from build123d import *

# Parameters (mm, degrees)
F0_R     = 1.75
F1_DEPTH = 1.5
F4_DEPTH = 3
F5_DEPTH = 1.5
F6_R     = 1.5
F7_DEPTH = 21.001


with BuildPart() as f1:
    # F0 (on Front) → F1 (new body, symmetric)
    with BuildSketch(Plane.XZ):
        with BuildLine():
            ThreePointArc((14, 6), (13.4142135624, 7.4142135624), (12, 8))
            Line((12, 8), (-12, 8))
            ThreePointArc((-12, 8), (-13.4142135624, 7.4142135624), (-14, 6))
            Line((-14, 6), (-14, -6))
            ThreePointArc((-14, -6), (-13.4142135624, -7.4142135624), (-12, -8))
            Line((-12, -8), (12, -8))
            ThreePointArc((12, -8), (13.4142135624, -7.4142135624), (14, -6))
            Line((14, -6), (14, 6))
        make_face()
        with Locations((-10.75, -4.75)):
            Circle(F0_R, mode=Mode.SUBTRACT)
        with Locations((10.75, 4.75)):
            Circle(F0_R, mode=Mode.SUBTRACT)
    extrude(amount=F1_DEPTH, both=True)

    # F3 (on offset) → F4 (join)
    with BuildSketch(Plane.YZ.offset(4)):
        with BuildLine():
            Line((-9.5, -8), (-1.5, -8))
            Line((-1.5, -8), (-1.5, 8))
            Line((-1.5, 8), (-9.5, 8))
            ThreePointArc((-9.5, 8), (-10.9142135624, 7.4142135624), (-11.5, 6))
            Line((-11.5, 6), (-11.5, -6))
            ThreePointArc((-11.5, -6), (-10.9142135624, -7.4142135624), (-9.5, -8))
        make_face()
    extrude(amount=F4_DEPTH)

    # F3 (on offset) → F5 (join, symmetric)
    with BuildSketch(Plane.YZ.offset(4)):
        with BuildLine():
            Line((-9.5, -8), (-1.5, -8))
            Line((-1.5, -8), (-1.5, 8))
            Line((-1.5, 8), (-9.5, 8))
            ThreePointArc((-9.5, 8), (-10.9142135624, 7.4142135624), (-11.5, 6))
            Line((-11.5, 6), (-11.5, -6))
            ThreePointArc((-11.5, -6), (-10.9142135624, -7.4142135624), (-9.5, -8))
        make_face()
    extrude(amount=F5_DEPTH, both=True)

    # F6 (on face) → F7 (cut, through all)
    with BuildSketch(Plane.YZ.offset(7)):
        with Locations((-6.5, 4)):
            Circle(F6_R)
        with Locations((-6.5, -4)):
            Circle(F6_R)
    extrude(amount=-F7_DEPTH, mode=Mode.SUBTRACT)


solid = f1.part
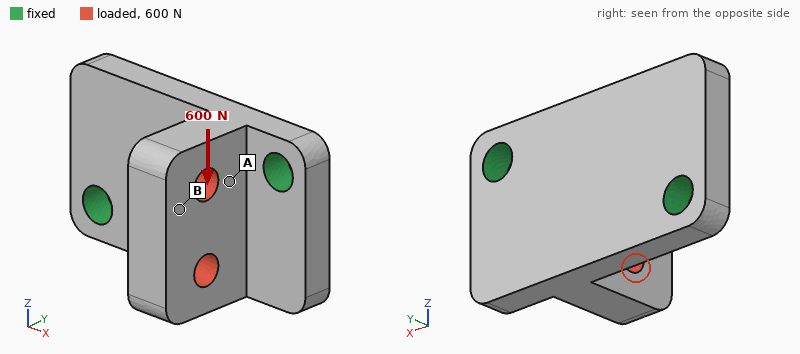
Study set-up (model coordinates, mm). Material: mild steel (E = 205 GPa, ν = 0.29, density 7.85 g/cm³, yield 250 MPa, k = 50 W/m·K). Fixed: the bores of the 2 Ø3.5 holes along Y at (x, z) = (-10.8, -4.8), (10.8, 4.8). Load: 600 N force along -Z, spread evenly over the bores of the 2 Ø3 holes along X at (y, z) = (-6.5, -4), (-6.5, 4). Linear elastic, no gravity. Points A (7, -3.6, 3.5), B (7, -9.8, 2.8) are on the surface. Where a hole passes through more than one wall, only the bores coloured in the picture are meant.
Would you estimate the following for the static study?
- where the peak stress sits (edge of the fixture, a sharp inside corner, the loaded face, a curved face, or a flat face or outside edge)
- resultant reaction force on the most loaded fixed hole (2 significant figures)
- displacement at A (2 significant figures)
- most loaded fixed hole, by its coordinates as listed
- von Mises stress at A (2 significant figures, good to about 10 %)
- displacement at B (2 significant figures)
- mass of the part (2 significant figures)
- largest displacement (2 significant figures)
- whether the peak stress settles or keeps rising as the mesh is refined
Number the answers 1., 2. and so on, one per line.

1. edge of the fixture
2. 460 N
3. 5.3 µm
4. (10.8, 4.8)
5. 44 MPa
6. 13 µm
7. 15 g
8. 19 µm
9. keeps rising
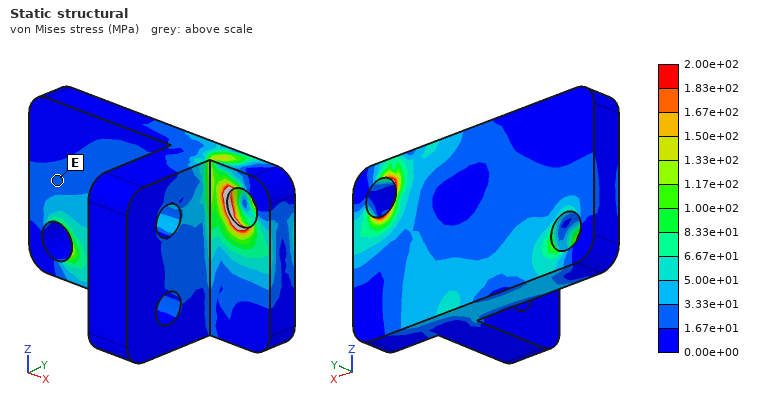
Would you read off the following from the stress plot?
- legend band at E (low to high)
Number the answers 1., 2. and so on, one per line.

1. 1.67e+01 to 3.33e+01 MPa
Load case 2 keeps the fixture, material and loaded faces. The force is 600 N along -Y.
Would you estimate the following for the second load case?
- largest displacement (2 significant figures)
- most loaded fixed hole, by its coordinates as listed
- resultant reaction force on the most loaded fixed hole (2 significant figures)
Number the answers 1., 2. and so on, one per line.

1. 10 µm
2. (10.8, 4.8)
3. 450 N
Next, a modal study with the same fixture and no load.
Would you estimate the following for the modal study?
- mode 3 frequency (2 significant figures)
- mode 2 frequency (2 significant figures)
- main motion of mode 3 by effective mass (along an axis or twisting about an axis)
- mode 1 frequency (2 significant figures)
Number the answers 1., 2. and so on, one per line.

1. 23 kHz
2. 15 kHz
3. along Y
4. 11 kHz
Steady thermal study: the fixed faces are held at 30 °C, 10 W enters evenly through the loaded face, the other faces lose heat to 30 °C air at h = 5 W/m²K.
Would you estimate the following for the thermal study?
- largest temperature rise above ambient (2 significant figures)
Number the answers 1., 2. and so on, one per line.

1. 41 K
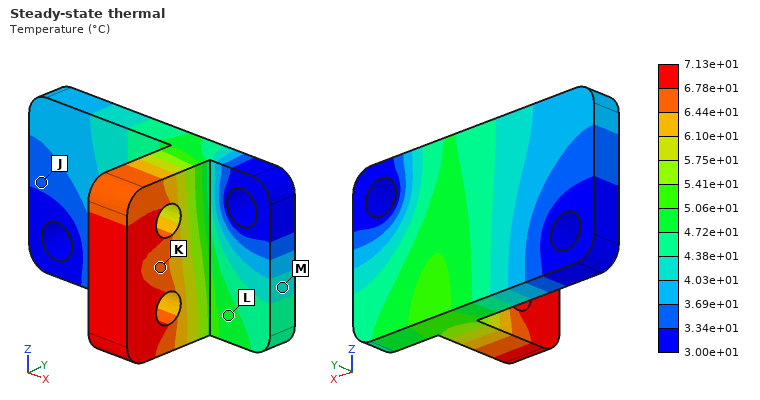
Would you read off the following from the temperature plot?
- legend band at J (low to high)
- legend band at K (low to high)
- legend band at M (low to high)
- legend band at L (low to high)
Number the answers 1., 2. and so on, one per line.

1. 3.34e+01 to 3.69e+01 °C
2. 6.44e+01 to 6.78e+01 °C
3. 4.03e+01 to 4.38e+01 °C
4. 4.72e+01 to 5.06e+01 °C
